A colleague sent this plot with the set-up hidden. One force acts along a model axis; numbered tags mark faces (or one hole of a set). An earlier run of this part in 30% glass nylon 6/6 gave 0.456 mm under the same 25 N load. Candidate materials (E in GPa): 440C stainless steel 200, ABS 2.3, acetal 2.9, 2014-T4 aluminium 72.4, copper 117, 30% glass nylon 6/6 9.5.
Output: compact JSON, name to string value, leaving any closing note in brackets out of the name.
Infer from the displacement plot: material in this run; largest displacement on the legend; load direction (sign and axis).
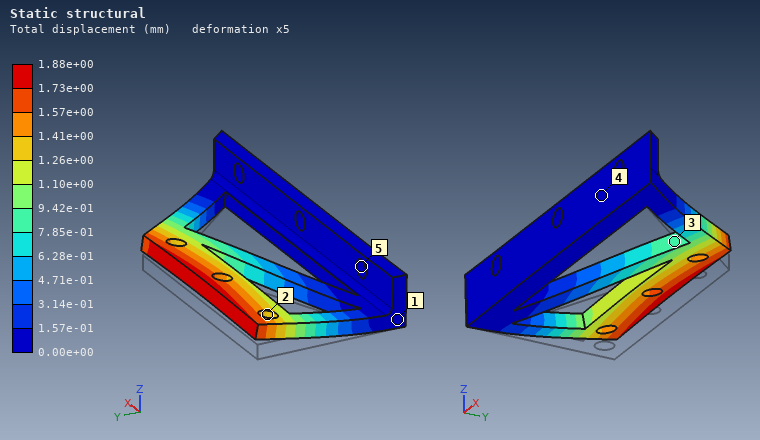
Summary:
{"material in this run": "ABS", "largest displacement on the legend": "1.88e+00 mm", "load direction": "+Z"}
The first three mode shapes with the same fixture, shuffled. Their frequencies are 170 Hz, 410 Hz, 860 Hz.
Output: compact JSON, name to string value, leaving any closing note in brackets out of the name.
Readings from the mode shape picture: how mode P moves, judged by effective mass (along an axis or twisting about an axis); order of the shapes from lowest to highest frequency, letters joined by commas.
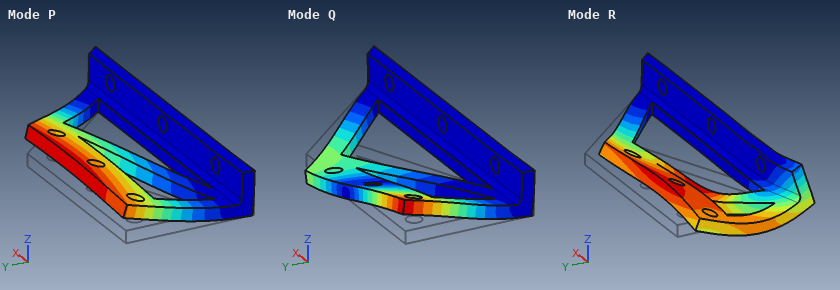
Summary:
{"how mode P moves, judged by effective mass": "along Z", "order of the shapes from lowest to highest frequency, letters joined by commas": "P, Q, R"}
